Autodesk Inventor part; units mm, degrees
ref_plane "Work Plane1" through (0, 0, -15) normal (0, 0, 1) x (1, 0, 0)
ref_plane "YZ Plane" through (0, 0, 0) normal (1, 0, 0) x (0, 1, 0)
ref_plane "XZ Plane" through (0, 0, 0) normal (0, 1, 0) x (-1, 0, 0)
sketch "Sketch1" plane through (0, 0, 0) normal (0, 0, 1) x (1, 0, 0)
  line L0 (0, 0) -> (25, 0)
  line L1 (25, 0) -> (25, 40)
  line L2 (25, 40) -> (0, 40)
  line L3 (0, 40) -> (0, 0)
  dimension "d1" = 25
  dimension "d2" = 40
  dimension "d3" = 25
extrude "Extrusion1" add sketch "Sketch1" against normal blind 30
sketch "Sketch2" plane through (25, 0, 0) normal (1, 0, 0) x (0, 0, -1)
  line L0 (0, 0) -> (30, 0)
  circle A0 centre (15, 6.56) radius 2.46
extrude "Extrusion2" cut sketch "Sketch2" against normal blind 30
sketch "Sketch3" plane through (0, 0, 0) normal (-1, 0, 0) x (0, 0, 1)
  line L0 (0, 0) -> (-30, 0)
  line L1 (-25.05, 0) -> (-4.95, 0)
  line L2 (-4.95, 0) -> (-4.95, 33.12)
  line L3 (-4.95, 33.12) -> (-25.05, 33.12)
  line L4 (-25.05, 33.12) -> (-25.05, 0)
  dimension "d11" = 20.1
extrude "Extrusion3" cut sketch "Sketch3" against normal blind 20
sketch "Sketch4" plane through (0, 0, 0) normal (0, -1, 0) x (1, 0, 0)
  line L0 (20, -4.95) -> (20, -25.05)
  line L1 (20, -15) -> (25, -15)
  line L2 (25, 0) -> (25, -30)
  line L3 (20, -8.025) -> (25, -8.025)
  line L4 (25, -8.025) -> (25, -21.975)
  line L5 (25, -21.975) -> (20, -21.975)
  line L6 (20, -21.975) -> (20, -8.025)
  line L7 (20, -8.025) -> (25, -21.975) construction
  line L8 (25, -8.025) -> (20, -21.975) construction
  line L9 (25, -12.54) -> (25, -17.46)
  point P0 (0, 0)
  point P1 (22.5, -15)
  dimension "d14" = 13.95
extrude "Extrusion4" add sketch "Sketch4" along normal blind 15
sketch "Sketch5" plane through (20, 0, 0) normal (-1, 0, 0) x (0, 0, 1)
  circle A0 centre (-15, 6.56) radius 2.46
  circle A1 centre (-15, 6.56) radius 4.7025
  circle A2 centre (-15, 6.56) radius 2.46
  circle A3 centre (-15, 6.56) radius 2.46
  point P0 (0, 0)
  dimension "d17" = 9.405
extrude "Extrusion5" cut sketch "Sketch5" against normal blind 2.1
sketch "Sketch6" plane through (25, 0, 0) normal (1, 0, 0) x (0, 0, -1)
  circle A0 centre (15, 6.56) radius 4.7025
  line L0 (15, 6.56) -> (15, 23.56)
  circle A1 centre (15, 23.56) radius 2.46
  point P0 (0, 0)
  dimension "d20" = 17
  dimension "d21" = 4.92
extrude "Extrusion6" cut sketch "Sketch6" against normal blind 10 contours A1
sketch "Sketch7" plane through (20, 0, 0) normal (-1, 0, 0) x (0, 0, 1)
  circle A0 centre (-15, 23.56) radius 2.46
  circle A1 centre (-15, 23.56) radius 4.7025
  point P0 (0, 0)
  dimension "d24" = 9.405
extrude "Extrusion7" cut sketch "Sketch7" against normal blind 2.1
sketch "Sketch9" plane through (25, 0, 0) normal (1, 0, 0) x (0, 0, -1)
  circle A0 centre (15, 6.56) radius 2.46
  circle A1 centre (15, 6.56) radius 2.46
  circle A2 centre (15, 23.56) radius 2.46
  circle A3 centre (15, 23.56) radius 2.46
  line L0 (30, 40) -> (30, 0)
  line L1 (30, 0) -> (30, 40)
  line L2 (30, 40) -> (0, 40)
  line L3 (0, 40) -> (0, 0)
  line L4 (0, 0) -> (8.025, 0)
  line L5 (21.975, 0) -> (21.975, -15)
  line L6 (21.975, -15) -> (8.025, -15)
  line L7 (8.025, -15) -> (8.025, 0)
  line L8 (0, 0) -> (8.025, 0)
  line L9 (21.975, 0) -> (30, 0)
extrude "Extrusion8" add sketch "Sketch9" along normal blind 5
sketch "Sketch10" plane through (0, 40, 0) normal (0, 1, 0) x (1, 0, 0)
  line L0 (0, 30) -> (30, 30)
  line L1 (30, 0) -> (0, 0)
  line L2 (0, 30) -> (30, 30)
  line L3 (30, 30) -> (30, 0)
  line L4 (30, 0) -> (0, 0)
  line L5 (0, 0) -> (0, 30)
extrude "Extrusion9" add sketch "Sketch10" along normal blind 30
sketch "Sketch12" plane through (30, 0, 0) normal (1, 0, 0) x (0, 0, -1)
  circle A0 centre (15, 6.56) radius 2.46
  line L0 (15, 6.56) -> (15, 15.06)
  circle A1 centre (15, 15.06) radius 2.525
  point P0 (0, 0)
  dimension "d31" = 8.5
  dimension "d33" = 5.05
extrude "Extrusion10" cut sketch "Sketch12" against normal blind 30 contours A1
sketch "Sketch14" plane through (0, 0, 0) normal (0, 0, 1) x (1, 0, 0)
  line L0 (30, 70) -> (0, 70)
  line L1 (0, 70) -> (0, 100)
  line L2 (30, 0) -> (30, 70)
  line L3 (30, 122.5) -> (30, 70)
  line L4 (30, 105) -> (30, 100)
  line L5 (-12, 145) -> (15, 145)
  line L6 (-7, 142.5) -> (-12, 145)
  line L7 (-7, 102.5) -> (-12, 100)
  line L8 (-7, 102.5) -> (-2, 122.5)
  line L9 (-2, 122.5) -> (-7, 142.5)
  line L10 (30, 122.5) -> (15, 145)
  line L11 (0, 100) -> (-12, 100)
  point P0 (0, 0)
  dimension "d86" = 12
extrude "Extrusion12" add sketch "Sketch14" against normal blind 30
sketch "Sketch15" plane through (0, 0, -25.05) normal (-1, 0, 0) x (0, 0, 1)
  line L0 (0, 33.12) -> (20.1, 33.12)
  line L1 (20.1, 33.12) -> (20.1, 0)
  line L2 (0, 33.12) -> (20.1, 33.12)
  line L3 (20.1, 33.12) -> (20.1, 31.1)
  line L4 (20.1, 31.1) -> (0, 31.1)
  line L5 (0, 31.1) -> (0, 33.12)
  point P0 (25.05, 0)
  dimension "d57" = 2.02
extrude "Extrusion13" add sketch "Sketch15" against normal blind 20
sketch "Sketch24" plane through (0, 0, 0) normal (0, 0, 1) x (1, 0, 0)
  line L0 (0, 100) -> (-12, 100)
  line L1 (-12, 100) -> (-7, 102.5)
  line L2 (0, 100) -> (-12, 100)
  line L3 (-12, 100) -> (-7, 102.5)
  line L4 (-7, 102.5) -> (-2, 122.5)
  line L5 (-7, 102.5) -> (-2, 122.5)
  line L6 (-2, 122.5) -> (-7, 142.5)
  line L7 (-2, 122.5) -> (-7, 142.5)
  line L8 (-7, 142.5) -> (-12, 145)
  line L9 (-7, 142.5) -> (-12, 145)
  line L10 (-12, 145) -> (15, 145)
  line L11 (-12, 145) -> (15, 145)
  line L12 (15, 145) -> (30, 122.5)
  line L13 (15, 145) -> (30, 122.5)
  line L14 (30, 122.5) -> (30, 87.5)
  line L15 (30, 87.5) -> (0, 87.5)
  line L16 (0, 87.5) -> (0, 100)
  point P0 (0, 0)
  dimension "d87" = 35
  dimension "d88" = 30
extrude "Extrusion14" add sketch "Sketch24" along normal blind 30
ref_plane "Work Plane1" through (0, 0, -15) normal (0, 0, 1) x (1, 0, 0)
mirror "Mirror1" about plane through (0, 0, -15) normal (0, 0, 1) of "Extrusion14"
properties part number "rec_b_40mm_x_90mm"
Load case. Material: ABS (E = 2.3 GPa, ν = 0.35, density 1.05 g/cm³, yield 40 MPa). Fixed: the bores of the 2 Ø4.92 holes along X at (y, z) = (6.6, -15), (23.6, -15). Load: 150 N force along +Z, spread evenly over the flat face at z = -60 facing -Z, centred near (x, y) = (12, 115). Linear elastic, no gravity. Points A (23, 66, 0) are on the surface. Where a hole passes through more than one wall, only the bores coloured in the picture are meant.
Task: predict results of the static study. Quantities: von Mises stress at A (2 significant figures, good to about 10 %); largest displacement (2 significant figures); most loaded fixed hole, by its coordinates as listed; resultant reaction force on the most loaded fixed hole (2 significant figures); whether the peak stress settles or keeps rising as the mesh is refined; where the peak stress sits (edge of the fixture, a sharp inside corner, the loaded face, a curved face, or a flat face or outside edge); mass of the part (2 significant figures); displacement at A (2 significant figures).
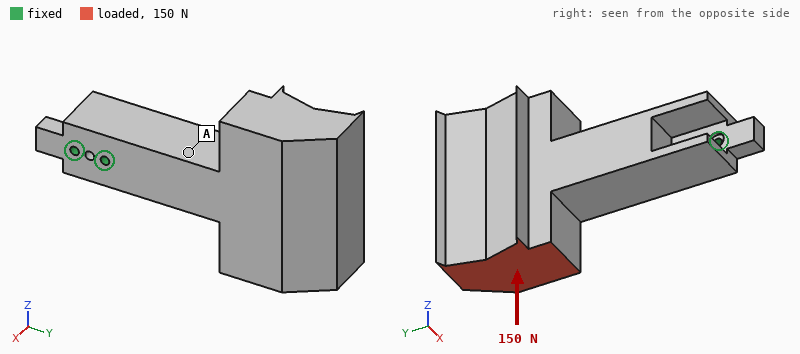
1.7 MPa
1.2 mm
(23.6, -15)
740 N
keeps rising
edge of the fixture
240 g
0.34 mm
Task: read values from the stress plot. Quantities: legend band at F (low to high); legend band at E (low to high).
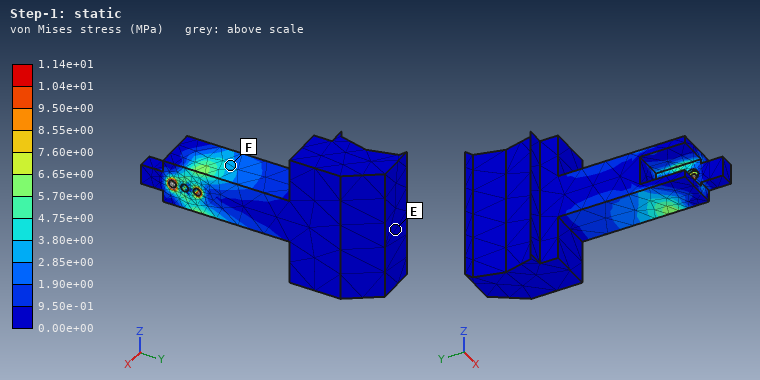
2.85e+00 to 3.80e+00 MPa
0.00e+00 to 9.50e-01 MPa
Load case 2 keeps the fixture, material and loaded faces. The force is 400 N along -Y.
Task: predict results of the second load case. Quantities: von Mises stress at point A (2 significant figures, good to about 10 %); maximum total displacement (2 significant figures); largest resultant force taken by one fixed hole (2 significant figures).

3.8 MPa
1.9 mm
850 N
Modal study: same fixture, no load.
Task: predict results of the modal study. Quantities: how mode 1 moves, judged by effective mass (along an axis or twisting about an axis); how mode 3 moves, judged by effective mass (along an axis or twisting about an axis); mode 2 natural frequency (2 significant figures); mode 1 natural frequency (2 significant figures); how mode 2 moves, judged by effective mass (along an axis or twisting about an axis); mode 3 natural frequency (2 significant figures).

along X
twisting about Y
160 Hz
140 Hz
along Z
300 Hz
